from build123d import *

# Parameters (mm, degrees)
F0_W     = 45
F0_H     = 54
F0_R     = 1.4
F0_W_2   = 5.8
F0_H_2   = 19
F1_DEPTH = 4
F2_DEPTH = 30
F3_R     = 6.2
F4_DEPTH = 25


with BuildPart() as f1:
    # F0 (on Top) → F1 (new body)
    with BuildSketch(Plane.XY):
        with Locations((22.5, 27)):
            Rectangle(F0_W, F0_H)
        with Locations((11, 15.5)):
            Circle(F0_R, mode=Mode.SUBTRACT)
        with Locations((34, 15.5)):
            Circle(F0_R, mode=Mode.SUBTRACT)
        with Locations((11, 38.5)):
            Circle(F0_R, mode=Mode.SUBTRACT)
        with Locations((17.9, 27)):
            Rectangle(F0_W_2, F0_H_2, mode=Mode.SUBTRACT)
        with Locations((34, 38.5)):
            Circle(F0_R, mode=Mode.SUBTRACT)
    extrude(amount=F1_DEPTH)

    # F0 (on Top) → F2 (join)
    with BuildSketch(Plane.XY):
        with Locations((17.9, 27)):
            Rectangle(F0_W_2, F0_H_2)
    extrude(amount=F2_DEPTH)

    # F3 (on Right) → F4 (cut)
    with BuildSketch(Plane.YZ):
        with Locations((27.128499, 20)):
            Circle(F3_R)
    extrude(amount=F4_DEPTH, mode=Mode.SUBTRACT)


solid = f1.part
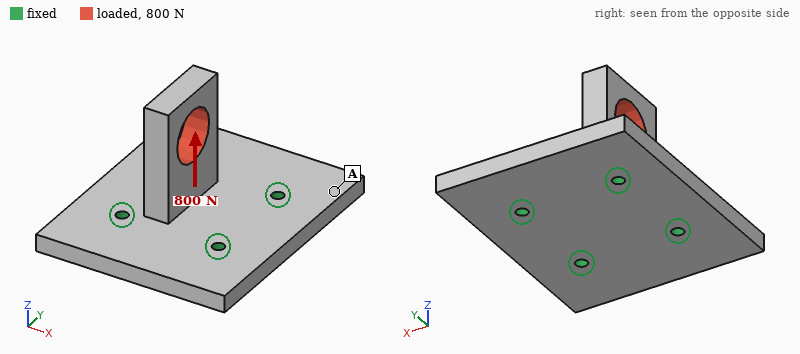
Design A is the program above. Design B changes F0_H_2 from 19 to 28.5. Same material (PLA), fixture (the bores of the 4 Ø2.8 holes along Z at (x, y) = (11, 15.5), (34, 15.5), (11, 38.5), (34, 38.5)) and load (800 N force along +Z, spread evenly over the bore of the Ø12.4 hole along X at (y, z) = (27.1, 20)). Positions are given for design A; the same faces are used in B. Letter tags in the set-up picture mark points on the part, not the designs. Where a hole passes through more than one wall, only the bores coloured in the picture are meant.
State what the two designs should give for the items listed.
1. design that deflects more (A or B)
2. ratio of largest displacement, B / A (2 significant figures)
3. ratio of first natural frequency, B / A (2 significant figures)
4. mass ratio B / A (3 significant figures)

A
0.75
0.98
1.12
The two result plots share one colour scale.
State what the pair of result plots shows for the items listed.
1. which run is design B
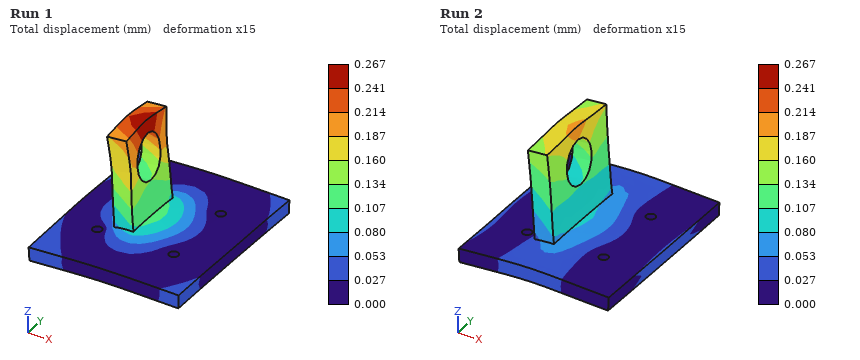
Run 2
